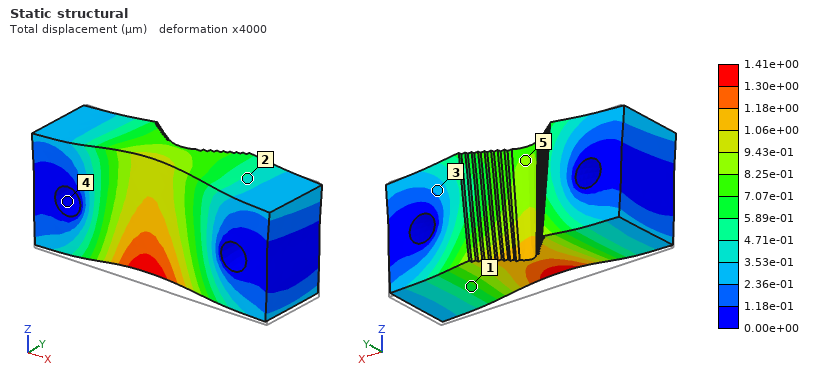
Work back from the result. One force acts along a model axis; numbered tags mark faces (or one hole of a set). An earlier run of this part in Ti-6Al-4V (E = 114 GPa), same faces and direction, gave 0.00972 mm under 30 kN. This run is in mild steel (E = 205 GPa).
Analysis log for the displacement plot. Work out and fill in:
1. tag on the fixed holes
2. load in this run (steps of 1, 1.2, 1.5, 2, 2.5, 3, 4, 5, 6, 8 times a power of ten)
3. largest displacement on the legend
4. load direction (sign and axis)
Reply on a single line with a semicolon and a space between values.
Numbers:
4; 8 kN; 1.41e+00 µm; +Z
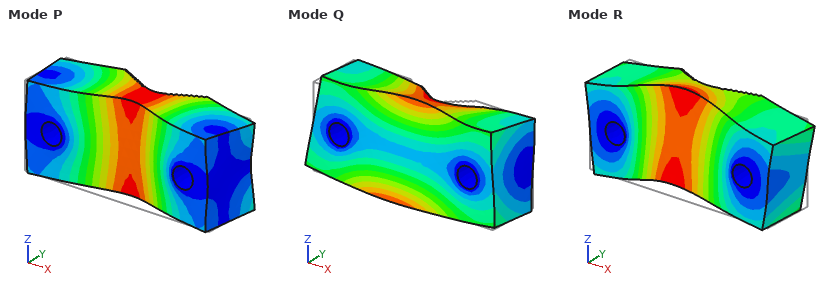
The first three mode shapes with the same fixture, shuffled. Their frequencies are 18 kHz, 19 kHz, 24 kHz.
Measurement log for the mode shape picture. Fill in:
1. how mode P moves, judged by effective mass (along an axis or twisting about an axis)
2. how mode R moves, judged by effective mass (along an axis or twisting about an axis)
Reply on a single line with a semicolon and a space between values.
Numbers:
along Y; along Z
